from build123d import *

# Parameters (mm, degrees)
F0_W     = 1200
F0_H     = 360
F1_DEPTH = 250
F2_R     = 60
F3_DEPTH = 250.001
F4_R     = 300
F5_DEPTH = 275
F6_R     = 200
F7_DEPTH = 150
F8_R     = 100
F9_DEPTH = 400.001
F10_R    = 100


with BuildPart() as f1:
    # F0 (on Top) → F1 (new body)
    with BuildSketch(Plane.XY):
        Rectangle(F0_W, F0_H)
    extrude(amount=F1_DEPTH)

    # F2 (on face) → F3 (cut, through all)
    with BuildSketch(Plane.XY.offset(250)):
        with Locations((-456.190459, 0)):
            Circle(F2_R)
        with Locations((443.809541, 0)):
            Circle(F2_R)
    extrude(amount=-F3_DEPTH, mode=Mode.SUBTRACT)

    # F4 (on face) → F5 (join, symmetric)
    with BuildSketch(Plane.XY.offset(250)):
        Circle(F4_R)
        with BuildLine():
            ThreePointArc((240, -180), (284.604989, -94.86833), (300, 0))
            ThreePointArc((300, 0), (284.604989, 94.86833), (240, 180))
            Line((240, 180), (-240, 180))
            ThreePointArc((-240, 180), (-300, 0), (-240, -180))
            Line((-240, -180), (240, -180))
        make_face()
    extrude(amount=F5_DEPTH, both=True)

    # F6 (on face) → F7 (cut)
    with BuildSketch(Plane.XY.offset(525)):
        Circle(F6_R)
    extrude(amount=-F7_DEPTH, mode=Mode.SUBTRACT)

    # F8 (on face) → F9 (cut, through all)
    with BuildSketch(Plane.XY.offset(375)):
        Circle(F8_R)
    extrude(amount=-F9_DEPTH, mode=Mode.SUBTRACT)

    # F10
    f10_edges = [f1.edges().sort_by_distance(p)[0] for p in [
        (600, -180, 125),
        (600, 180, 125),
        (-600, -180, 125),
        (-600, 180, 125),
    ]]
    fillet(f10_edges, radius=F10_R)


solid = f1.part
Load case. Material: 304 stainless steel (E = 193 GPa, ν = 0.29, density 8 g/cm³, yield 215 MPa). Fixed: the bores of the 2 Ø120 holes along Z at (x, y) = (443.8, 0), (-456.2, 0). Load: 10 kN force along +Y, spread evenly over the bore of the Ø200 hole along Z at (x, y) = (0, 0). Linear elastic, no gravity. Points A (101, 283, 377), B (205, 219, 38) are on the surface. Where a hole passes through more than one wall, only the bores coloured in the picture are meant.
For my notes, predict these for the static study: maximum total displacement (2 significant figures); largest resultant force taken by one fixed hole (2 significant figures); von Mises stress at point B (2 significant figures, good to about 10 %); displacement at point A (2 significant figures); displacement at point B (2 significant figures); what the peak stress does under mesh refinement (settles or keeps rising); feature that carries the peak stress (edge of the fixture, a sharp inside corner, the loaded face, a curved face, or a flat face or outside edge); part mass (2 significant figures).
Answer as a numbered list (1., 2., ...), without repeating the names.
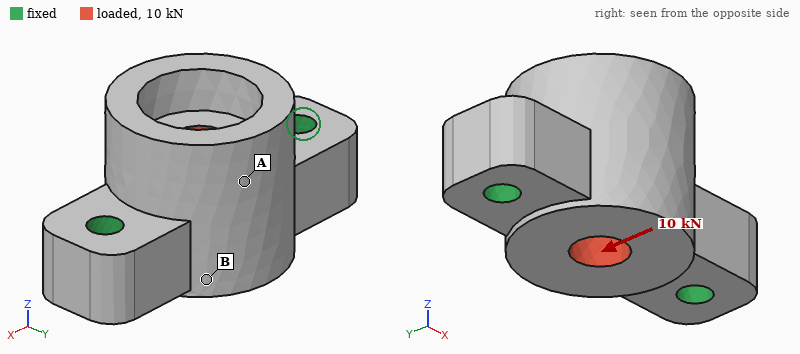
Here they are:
1. 0.58 µm
2. 5.1 kN
3. 0.089 MPa
4. 0.50 µm
5. 0.24 µm
6. keeps rising
7. edge of the fixture
8. 1400 kg
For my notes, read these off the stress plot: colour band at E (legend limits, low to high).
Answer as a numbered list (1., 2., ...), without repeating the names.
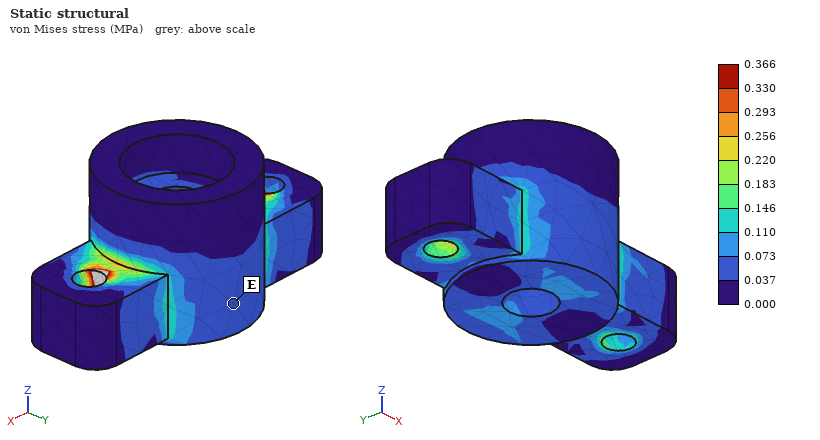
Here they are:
1. 0.037 to 0.073 MPa
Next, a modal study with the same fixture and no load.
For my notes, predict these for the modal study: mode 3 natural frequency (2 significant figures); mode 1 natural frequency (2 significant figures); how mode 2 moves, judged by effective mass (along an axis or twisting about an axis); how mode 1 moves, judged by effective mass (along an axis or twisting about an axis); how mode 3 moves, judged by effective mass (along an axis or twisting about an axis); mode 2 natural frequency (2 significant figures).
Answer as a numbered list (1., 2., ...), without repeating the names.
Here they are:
1. 1100 Hz
2. 540 Hz
3. along Z
4. along Y
5. along Y
6. 870 Hz
